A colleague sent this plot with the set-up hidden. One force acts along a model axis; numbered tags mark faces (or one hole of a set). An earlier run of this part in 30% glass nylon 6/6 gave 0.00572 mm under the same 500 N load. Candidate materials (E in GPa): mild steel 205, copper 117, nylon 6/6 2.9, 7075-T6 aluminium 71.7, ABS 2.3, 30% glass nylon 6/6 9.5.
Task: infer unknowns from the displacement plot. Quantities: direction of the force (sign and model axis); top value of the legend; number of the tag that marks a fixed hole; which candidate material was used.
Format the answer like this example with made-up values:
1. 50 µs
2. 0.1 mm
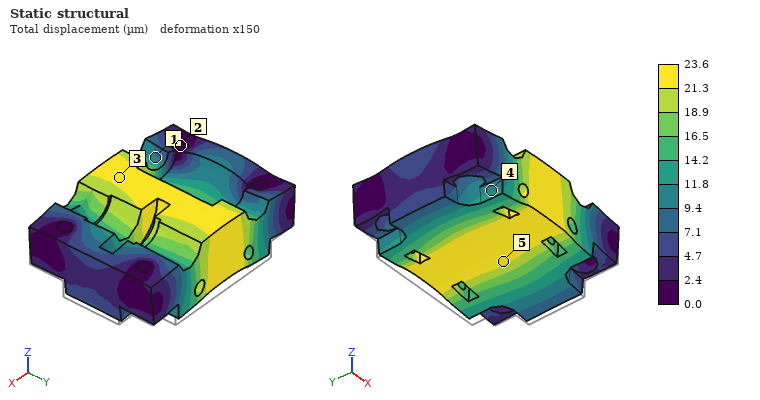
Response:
1. +Z
2. 23.6 µm
3. 2
4. ABS
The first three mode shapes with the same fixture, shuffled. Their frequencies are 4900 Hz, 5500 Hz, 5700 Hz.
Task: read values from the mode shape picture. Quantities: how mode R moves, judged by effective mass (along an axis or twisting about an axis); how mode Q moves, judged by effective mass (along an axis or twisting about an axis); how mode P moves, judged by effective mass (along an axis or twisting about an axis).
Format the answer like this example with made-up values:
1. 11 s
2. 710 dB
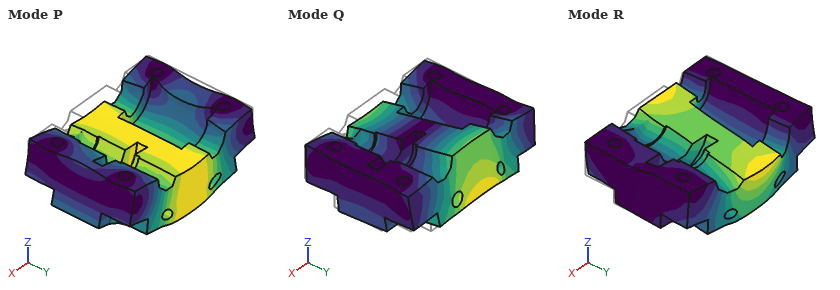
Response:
1. along Y
2. along Y
3. along Z
